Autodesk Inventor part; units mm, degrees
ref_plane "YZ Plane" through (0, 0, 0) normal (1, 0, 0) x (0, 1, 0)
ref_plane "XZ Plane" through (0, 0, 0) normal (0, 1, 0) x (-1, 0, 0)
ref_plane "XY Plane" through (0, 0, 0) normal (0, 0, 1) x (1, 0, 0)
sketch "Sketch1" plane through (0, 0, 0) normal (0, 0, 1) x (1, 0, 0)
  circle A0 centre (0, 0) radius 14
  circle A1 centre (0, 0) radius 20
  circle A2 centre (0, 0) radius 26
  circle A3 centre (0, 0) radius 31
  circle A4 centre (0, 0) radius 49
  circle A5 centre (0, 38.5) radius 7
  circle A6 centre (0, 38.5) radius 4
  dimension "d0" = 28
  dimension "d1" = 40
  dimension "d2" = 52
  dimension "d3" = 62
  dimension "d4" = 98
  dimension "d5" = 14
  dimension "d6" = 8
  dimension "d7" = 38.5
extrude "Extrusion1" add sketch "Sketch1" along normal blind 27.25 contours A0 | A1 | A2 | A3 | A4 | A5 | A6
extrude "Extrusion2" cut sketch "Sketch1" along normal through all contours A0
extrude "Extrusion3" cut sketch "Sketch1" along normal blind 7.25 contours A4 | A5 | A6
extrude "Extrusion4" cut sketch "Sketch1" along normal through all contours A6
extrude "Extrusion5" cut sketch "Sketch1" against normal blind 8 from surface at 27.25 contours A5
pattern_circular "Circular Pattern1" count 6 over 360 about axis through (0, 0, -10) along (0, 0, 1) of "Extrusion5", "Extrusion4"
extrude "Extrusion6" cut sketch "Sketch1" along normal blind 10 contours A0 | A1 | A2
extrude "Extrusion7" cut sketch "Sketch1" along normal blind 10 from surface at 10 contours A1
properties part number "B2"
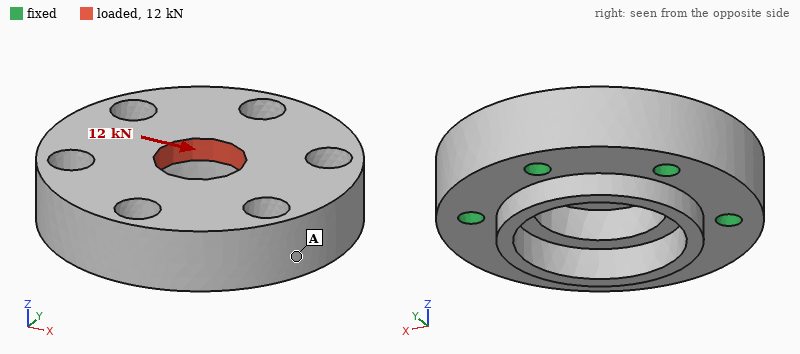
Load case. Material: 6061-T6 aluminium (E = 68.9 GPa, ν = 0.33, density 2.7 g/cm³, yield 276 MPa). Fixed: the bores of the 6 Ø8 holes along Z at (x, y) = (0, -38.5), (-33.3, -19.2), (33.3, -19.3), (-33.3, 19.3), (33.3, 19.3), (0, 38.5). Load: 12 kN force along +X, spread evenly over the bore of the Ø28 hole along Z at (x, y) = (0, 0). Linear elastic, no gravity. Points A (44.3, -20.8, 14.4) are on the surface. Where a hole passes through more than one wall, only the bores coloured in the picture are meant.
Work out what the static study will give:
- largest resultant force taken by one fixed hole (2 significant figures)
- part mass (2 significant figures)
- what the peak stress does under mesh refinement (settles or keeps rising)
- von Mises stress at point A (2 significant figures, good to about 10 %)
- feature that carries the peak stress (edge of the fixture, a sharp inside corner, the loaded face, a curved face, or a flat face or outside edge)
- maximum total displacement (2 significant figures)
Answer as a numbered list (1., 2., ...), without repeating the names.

1. 2.5 kN
2. 330 g
3. keeps rising
4. 5.6 MPa
5. edge of the fixture
6. 10 µm
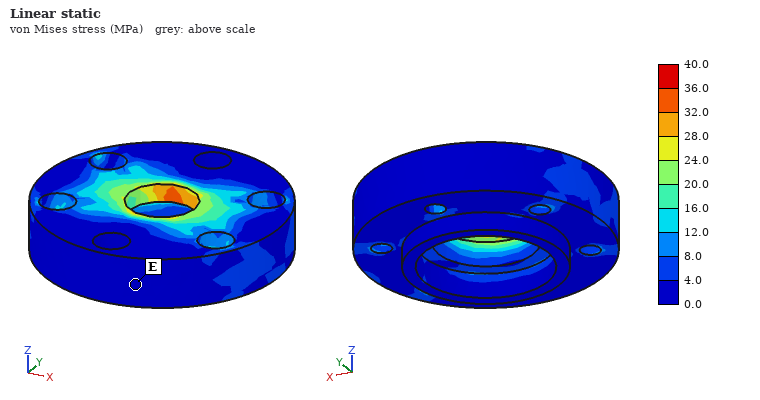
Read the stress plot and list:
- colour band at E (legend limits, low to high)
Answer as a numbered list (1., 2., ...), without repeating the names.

1. 0.0 to 4.0 MPa
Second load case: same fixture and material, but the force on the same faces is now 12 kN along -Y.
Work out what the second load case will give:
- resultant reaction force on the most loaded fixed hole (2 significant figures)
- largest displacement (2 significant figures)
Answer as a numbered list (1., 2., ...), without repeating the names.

1. 2.8 kN
2. 10 µm
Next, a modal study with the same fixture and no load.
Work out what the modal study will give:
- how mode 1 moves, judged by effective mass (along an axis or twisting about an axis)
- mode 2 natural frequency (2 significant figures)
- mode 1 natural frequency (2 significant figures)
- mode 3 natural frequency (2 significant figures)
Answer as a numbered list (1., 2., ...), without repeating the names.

1. along Z
2. 23 kHz
3. 21 kHz
4. 23 kHz
